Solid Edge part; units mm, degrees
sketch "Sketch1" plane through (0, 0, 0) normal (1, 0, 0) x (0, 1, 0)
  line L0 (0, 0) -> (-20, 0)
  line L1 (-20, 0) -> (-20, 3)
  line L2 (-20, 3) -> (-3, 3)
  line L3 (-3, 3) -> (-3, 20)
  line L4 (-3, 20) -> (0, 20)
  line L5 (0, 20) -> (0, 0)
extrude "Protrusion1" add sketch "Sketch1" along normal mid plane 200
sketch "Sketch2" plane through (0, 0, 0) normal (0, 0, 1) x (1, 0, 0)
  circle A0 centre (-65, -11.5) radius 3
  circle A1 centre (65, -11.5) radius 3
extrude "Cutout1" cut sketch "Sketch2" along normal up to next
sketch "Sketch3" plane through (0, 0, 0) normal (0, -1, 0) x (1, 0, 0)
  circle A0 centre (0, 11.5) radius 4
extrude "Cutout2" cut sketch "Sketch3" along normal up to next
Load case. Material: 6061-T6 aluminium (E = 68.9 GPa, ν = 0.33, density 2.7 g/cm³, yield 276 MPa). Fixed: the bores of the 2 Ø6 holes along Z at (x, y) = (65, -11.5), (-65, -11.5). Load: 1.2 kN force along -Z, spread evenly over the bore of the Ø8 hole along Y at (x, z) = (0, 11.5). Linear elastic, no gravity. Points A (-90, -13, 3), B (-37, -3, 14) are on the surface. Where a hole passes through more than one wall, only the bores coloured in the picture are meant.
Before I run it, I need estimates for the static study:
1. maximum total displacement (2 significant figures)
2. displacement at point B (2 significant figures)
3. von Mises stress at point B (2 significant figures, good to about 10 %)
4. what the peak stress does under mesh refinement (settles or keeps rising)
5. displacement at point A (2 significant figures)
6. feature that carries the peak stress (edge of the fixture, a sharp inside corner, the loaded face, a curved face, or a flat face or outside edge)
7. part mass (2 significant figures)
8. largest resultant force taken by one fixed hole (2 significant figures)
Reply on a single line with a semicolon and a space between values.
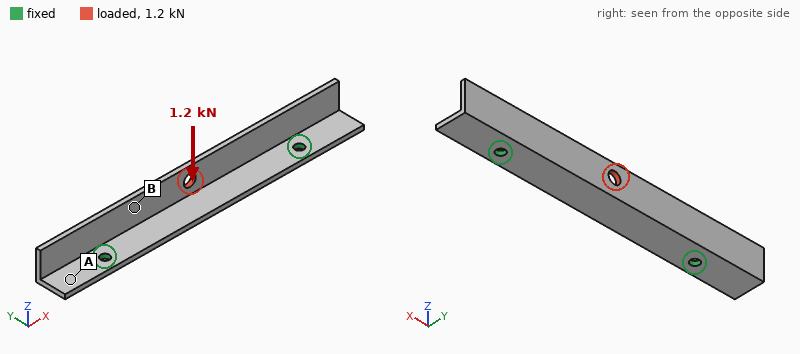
0.32 mm; 0.18 mm; 31 MPa; keeps rising; 0.066 mm; edge of the fixture; 59 g; 1.1 kN
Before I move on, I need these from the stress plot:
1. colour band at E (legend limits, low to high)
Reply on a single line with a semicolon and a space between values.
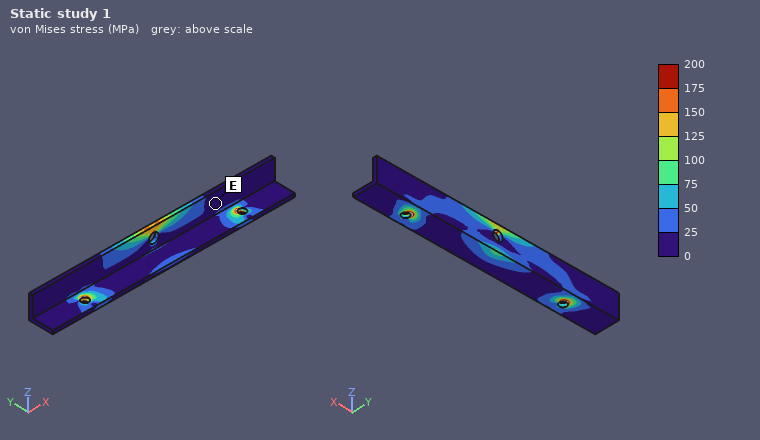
0 to 25 MPa
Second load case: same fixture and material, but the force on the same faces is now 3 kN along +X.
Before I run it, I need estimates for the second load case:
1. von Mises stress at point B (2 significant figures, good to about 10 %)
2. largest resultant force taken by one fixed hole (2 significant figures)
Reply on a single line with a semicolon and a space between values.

15 MPa; 1.5 kN
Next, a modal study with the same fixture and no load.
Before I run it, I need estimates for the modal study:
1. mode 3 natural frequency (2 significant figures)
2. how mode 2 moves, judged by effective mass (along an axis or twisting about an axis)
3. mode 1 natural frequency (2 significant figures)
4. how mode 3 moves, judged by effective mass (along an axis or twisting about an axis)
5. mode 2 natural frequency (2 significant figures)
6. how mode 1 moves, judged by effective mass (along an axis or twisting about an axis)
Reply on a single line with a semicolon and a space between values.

3200 Hz; along Z; 2000 Hz; twisting about Z; 2400 Hz; along Y
